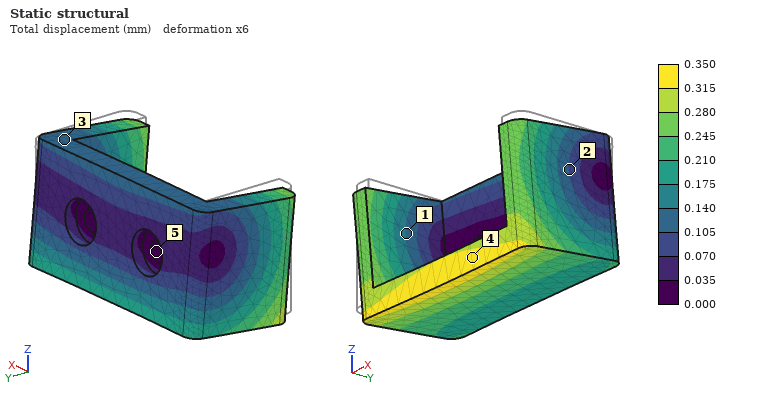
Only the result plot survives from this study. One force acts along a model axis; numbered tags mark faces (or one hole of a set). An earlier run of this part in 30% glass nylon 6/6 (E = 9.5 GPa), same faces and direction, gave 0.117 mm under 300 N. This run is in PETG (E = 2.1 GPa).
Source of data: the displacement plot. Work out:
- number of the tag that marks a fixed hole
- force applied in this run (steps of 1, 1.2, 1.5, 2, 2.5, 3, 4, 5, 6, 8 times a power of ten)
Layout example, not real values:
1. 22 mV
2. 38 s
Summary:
1. 5
2. 200 N
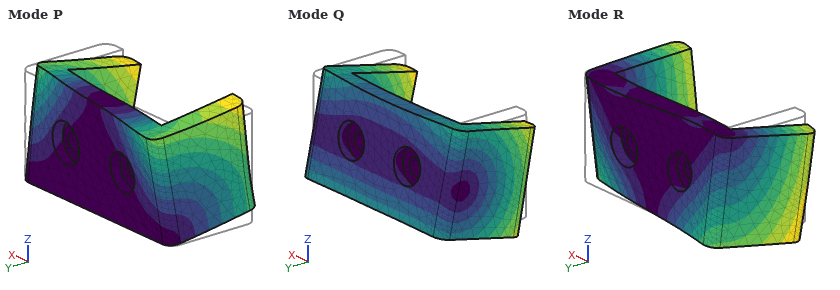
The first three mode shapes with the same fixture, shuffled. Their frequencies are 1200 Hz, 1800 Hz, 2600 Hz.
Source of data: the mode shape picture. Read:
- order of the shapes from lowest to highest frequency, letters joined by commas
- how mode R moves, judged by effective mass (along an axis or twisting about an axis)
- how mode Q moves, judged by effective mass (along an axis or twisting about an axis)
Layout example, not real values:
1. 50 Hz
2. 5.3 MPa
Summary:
1. Q, R, P
2. along X
3. along Z
